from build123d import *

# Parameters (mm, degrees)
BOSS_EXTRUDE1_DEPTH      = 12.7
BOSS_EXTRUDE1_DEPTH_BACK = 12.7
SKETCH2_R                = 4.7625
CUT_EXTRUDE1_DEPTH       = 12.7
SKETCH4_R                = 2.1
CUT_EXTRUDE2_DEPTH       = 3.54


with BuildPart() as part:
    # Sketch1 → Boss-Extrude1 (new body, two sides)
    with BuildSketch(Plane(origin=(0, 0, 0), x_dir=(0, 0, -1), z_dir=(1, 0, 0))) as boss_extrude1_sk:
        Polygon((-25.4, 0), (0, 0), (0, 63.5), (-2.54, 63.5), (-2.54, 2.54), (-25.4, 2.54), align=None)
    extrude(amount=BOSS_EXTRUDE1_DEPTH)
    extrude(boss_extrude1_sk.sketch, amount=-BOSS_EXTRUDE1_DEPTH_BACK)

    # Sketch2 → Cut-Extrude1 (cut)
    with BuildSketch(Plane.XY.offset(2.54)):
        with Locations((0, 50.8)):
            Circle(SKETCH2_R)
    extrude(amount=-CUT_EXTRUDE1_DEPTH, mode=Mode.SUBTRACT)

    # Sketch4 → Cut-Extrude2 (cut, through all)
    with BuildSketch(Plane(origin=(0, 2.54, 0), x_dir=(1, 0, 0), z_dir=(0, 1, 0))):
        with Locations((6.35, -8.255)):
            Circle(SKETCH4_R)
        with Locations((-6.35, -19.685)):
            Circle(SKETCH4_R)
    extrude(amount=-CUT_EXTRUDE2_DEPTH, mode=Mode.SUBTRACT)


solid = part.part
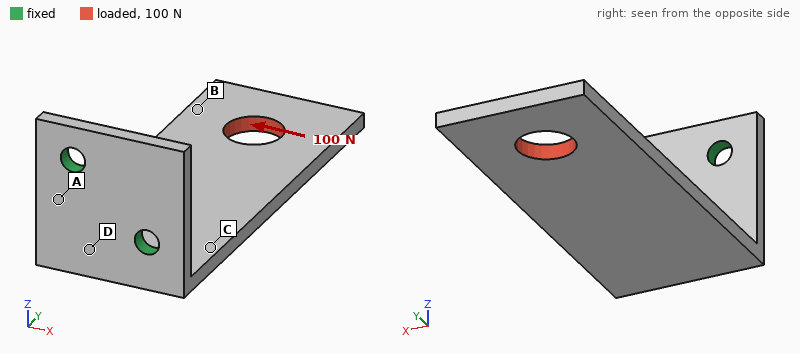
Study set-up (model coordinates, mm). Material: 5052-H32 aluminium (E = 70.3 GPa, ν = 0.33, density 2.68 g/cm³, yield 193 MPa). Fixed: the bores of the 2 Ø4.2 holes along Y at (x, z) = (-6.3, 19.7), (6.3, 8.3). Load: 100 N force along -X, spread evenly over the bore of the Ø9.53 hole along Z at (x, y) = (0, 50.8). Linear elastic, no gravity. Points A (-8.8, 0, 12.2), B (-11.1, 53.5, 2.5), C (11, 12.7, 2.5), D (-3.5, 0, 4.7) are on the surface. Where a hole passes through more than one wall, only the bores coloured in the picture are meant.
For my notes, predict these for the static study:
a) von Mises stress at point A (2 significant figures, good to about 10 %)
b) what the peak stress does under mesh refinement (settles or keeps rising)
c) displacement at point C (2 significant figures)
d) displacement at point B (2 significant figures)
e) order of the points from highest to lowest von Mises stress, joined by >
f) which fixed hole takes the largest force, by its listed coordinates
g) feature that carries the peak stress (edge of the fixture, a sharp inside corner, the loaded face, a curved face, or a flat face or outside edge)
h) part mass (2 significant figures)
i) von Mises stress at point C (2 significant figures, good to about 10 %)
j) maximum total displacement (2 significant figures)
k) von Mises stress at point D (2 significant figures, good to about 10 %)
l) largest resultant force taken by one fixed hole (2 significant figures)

62 MPa
keeps rising
0.086 mm
0.42 mm
A > D > C > B
(6.3, 8.3)
edge of the fixture
14 g
28 MPa
0.50 mm
42 MPa
140 N
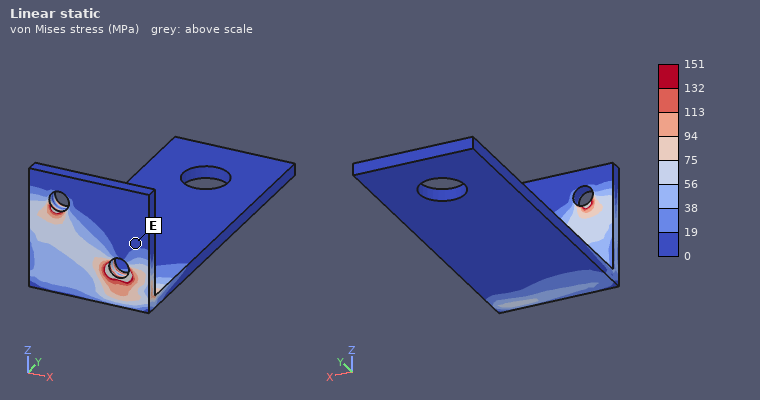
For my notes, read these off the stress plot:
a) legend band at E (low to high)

0 to 19 MPa
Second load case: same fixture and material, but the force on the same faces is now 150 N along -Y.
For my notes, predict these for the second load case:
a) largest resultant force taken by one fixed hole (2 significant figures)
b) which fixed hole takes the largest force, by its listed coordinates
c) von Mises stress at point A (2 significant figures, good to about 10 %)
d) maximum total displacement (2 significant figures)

140 N
(6.3, 8.3)
16 MPa
0.15 mm
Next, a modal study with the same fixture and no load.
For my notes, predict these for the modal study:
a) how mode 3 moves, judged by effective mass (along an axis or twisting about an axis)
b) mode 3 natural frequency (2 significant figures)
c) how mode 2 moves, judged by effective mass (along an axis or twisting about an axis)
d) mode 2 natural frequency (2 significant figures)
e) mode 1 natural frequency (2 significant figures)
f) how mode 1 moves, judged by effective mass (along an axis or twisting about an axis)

twisting about Y
2600 Hz
along X
1200 Hz
490 Hz
along Z
